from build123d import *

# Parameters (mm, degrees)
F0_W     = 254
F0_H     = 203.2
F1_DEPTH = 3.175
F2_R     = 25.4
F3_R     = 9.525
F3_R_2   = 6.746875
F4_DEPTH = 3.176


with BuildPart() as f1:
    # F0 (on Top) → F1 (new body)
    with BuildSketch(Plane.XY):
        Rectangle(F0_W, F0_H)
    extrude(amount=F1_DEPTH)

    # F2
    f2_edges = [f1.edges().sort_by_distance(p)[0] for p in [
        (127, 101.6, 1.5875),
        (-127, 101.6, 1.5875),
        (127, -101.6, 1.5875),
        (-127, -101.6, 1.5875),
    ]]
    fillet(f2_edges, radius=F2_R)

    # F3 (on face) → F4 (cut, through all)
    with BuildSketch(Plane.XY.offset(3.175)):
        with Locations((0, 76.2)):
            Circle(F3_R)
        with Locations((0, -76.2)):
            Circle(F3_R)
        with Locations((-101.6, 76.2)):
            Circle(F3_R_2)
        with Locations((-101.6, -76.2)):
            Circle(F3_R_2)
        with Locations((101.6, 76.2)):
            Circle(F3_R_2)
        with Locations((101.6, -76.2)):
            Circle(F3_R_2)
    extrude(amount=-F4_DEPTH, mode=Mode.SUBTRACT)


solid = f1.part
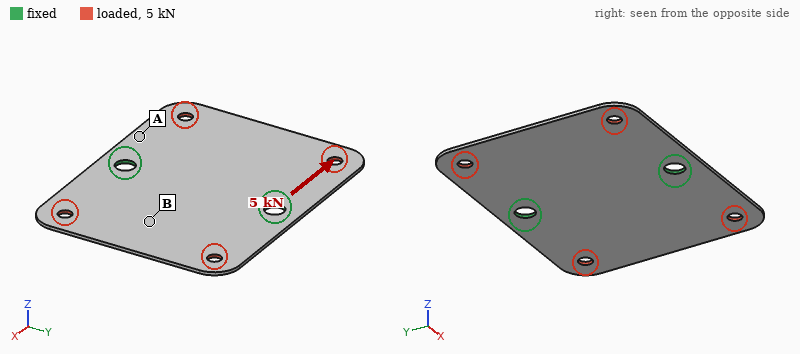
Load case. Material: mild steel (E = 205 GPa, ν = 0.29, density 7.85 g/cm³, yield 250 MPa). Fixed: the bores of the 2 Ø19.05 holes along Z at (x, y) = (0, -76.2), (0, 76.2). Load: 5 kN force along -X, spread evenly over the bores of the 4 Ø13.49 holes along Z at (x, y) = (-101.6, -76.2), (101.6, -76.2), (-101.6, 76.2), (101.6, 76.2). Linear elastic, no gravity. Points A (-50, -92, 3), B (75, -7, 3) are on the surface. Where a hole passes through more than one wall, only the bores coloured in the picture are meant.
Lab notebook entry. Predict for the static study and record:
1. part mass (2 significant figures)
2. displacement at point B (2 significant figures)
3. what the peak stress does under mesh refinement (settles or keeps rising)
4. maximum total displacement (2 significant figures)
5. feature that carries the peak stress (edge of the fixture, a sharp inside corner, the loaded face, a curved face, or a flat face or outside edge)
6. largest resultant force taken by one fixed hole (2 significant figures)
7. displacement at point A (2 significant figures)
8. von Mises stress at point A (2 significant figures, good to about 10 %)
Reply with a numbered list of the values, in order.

1. 1.2 kg
2. 1.9 µm
3. keeps rising
4. 4.5 µm
5. edge of the fixture
6. 2.5 kN
7. 1.9 µm
8. 7.3 MPa
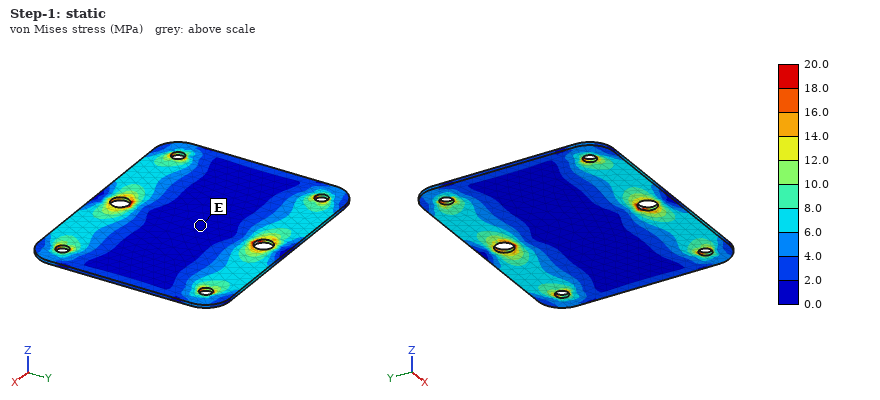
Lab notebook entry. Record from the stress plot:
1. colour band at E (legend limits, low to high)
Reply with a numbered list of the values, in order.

1. 0.0 to 2.0 MPa
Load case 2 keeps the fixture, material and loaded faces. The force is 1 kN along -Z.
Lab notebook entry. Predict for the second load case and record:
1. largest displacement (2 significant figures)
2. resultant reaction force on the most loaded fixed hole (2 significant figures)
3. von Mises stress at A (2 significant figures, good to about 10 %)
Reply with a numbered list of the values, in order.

1. 1.9 mm
2. 500 N
3. 81 MPa
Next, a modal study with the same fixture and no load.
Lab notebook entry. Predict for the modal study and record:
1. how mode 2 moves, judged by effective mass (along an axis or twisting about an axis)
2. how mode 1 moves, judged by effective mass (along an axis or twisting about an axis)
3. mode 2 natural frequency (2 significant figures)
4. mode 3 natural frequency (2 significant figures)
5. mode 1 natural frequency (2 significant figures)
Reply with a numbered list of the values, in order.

1. along Z
2. twisting about Y
3. 180 Hz
4. 330 Hz
5. 160 Hz
